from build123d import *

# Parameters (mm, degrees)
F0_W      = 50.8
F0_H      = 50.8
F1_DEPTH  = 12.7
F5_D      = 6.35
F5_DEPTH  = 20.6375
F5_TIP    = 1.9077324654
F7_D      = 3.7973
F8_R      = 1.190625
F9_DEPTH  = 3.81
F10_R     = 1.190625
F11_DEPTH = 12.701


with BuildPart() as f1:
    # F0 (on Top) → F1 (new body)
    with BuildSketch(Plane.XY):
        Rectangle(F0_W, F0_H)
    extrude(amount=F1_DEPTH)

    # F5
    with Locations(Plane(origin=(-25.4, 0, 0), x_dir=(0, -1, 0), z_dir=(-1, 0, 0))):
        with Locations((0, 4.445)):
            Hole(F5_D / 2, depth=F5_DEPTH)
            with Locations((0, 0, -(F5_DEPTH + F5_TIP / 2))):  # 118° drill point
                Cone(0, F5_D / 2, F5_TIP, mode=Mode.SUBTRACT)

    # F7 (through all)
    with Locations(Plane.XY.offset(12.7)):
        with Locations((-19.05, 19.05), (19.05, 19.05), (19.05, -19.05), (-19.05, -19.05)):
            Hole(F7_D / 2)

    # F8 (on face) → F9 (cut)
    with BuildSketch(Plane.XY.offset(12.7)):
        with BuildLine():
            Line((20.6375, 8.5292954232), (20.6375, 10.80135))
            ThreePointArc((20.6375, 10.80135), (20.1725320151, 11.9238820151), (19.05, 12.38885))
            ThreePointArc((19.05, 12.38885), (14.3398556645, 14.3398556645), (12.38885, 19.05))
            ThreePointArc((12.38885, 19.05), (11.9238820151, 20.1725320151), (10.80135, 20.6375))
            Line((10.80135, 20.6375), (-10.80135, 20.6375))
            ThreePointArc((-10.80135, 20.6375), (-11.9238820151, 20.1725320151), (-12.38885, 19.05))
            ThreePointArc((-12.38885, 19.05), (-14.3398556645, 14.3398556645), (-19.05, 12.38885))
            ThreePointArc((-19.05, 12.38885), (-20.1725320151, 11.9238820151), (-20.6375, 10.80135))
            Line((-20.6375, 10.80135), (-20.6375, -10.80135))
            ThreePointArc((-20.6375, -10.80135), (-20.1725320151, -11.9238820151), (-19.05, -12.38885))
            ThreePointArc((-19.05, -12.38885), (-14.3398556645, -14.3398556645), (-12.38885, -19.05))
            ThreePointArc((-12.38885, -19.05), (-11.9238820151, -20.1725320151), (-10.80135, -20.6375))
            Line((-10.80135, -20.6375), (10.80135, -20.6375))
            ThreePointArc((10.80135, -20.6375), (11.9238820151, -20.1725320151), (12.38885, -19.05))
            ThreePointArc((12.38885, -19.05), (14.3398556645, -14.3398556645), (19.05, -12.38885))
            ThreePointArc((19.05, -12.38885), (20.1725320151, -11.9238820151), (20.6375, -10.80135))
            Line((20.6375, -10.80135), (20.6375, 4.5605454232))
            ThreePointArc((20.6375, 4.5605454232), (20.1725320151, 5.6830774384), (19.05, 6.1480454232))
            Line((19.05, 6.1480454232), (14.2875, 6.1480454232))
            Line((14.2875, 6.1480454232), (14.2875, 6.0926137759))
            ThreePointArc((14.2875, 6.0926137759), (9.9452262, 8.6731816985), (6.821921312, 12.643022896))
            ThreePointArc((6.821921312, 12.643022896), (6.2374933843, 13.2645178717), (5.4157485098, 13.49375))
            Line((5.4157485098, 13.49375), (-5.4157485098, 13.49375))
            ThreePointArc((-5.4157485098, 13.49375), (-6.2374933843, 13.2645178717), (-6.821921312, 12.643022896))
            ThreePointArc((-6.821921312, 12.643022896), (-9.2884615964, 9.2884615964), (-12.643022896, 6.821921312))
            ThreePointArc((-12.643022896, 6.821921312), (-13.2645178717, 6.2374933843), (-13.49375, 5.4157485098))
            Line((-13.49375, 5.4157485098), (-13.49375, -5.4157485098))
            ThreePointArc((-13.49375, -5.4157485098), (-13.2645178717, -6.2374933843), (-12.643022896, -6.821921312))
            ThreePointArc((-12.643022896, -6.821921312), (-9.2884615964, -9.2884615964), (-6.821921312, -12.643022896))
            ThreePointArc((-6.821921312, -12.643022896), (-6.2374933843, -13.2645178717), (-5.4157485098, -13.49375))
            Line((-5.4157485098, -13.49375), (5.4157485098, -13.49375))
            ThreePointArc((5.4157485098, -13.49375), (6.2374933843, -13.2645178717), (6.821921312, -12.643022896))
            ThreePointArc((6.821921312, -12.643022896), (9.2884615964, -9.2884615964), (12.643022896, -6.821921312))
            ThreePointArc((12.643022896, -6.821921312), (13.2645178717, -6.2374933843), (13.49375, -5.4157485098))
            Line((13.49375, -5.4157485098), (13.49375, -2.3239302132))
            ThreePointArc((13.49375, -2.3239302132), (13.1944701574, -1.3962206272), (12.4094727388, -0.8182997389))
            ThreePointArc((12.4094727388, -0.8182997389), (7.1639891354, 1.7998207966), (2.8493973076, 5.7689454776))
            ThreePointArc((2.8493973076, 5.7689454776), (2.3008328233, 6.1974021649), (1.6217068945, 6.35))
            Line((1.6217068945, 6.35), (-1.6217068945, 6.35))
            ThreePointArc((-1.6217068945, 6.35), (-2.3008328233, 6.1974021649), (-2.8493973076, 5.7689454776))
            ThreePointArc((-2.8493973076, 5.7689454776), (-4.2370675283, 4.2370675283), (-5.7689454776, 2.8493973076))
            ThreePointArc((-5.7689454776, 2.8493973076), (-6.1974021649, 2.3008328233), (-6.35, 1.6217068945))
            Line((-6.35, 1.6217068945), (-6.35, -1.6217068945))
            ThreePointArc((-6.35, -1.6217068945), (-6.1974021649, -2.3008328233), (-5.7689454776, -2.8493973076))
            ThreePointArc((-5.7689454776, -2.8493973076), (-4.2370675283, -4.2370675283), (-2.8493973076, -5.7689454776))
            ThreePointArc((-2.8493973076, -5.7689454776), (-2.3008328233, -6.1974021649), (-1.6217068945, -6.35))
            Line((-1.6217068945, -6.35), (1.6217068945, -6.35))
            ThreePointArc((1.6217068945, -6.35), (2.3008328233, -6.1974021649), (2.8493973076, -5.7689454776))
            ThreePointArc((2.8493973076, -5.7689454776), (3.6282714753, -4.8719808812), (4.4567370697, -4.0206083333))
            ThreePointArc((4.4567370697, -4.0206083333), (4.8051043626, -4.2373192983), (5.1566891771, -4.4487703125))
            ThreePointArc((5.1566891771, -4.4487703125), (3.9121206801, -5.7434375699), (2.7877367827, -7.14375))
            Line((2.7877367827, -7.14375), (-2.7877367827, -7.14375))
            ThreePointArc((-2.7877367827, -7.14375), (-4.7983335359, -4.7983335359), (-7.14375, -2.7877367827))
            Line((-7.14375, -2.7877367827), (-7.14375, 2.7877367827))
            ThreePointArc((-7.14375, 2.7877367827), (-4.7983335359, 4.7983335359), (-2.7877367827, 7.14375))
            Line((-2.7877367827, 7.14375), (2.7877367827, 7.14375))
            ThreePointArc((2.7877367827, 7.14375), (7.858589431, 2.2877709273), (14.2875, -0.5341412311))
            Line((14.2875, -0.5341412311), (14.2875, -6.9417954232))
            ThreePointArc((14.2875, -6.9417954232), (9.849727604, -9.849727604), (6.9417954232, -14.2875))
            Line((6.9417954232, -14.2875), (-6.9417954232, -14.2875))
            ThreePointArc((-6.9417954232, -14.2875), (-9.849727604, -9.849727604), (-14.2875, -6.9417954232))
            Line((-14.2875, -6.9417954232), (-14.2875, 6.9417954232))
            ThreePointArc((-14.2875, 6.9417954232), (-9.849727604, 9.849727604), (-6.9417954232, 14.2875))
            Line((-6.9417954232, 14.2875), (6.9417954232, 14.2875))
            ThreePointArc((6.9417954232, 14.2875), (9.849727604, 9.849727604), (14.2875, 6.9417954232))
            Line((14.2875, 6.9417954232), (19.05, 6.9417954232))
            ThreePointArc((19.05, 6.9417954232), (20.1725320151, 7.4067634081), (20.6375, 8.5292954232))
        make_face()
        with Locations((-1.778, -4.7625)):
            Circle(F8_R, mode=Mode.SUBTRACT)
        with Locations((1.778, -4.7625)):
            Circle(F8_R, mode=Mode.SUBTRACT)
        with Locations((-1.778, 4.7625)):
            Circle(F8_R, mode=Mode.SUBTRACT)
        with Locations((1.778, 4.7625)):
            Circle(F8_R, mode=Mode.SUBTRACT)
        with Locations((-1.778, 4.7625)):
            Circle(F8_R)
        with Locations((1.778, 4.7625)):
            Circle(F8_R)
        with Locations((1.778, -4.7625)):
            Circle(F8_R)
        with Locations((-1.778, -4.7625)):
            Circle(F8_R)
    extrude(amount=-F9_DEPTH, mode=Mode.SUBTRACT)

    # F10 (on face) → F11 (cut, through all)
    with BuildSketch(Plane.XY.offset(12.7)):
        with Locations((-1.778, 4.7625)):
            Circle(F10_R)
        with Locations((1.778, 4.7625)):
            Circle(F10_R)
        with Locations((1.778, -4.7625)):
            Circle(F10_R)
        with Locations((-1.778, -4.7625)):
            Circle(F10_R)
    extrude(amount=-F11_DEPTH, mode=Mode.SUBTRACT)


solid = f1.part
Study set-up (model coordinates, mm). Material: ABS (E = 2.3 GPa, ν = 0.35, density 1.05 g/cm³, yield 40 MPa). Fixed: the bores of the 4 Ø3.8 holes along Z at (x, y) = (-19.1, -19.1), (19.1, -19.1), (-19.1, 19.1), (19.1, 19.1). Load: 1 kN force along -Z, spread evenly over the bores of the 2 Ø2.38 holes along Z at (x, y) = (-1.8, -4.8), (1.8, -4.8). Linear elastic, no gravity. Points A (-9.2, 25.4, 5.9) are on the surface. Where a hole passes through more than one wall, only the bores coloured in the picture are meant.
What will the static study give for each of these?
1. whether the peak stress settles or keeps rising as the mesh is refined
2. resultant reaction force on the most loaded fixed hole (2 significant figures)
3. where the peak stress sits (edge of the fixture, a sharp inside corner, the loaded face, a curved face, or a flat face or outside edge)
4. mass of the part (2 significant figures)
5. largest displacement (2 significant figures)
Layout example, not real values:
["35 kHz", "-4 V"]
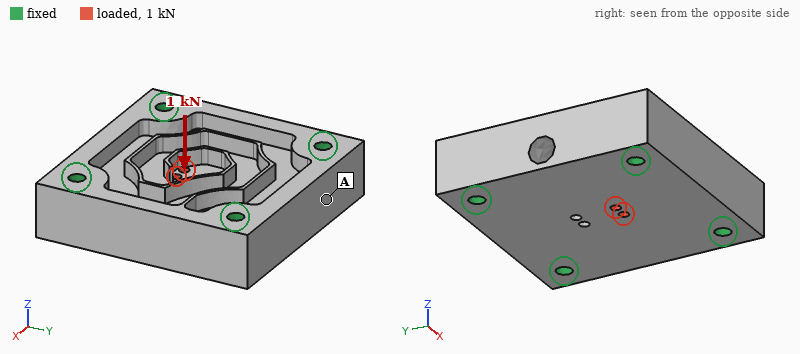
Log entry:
["keeps rising", "330 N", "a sharp inside corner", "28 g", "0.21 mm"]
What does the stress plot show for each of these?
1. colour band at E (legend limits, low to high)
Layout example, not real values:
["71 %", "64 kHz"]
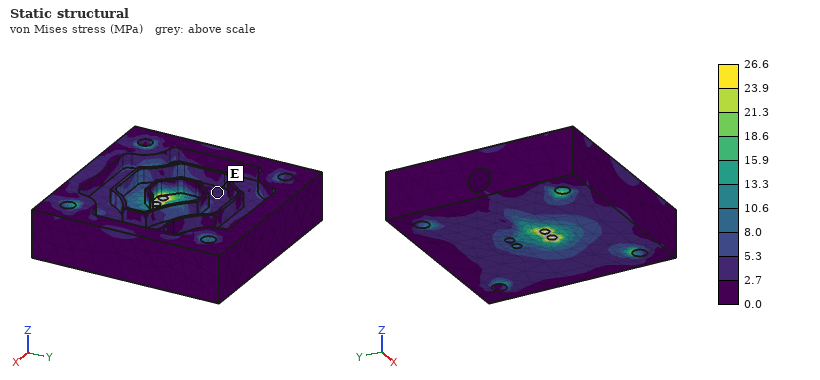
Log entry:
["2.7 to 5.3 MPa"]
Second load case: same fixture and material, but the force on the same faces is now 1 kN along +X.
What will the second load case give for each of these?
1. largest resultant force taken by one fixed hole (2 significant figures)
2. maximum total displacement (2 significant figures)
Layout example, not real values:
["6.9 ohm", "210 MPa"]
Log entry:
["350 N", "61 µm"]
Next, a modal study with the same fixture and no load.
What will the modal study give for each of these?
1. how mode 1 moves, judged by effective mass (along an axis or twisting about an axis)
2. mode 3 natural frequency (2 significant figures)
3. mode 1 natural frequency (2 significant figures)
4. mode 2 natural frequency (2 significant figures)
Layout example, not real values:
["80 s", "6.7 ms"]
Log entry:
["along Z", "8700 Hz", "5900 Hz", "8500 Hz"]
